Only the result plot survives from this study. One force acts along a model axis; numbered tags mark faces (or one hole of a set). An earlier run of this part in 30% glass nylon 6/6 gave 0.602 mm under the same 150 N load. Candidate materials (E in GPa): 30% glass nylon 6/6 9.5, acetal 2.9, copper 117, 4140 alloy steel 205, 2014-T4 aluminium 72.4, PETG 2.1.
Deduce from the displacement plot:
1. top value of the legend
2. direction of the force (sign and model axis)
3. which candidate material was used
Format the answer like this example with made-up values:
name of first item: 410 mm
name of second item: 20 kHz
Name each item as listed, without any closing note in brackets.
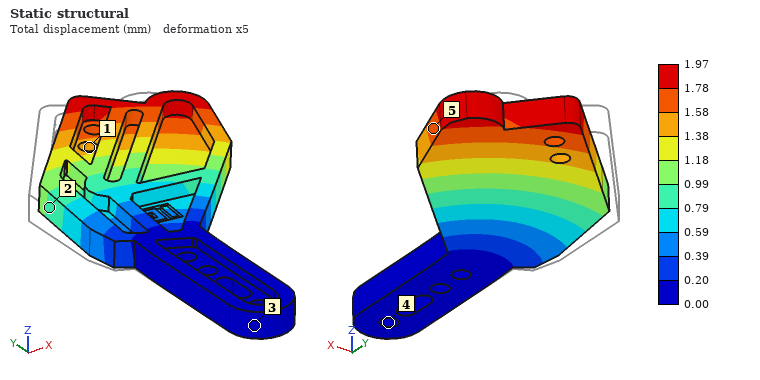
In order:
top value of the legend: 1.97 mm
direction of the force: +X
which candidate material was used: acetal
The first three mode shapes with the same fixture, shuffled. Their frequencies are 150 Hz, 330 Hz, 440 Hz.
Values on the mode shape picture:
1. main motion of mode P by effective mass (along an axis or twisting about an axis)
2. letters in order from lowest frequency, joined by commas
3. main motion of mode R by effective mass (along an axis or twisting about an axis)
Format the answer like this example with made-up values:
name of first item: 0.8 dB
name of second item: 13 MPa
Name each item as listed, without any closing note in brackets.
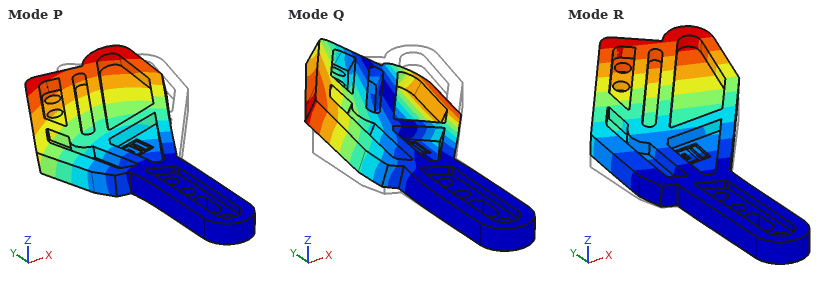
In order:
main motion of mode P by effective mass: along X
letters in order from lowest frequency, joined by commas: R, P, Q
main motion of mode R by effective mass: along Z
